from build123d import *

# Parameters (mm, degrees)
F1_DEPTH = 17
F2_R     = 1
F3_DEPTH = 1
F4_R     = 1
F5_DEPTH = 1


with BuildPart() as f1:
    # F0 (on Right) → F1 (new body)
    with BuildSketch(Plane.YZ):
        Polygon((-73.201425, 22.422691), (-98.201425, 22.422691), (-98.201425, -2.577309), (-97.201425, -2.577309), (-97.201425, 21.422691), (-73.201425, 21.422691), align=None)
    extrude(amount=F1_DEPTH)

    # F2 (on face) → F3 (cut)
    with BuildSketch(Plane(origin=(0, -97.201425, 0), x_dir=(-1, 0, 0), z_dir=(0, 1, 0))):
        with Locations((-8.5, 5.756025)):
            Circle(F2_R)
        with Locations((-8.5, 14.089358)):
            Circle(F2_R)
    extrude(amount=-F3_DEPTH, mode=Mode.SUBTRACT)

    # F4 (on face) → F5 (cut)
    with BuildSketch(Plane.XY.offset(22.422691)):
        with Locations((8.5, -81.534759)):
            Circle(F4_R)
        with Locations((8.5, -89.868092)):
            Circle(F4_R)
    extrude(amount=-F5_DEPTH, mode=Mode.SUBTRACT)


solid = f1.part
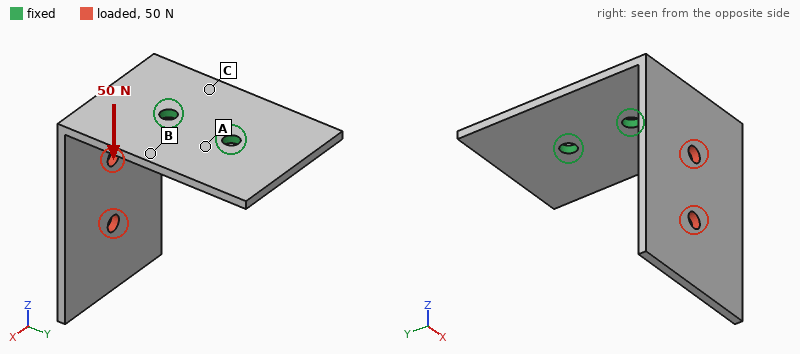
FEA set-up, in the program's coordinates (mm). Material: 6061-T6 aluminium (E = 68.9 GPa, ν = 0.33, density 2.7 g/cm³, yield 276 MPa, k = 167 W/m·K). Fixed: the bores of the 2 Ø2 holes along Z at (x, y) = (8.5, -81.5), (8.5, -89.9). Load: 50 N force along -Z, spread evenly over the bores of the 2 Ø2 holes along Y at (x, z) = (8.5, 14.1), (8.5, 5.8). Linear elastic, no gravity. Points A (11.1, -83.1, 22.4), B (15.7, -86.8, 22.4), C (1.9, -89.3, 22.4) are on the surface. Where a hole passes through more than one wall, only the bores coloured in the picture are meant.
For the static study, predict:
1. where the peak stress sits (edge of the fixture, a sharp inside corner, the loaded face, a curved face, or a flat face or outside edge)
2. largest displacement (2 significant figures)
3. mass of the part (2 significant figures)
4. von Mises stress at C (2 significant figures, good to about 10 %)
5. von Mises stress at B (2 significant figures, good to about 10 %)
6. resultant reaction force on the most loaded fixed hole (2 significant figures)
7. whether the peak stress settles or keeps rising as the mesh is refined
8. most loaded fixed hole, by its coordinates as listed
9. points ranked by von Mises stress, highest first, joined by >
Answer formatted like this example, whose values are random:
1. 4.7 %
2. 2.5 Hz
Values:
1. edge of the fixture
2. 0.41 mm
3. 2.2 g
4. 51 MPa
5. 29 MPa
6. 65 N
7. keeps rising
8. (8.5, -89.9)
9. C > B > A
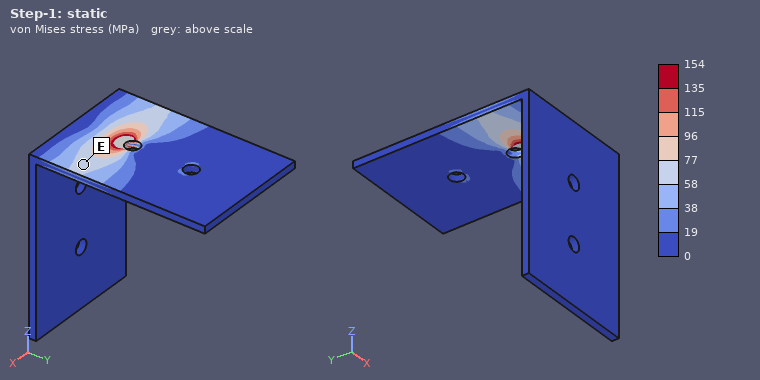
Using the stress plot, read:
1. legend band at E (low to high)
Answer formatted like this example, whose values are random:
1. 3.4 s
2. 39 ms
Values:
1. 58 to 77 MPa
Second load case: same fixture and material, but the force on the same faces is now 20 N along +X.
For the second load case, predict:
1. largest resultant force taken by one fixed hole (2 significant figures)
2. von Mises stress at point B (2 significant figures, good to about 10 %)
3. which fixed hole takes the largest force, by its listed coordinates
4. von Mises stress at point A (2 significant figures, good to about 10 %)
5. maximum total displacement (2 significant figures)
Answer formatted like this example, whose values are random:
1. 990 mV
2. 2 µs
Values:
1. 34 N
2. 34 MPa
3. (8.5, -89.9)
4. 14 MPa
5. 0.28 mm
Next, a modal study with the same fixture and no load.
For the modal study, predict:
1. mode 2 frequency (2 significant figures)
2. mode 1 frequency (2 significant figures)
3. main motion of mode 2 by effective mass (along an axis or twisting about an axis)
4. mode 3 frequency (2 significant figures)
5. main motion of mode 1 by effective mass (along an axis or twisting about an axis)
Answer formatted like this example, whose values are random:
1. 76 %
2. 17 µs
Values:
1. 1500 Hz
2. 910 Hz
3. along X
4. 4100 Hz
5. along Y
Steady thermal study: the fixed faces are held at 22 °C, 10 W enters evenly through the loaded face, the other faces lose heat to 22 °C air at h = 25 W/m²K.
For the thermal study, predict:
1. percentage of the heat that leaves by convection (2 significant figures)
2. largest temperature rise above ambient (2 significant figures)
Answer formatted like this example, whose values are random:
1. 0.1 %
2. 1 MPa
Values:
1. 14 %
2. 73 K
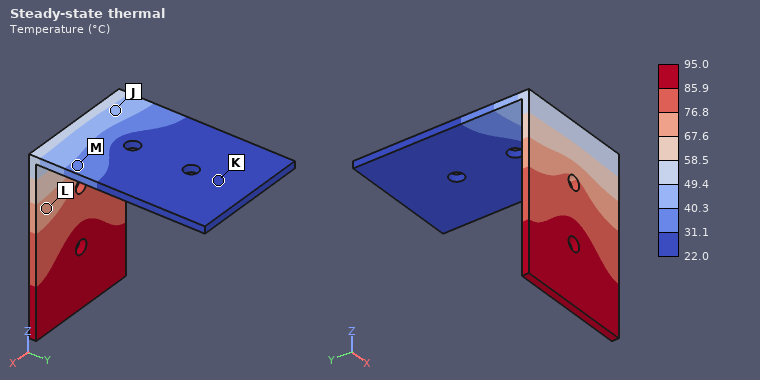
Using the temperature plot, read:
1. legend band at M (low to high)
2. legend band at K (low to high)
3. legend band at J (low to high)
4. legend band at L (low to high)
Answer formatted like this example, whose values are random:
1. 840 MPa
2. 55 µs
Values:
1. 31.1 to 40.3 °C
2. 22.0 to 31.1 °C
3. 40.3 to 49.4 °C
4. 67.6 to 76.8 °C
